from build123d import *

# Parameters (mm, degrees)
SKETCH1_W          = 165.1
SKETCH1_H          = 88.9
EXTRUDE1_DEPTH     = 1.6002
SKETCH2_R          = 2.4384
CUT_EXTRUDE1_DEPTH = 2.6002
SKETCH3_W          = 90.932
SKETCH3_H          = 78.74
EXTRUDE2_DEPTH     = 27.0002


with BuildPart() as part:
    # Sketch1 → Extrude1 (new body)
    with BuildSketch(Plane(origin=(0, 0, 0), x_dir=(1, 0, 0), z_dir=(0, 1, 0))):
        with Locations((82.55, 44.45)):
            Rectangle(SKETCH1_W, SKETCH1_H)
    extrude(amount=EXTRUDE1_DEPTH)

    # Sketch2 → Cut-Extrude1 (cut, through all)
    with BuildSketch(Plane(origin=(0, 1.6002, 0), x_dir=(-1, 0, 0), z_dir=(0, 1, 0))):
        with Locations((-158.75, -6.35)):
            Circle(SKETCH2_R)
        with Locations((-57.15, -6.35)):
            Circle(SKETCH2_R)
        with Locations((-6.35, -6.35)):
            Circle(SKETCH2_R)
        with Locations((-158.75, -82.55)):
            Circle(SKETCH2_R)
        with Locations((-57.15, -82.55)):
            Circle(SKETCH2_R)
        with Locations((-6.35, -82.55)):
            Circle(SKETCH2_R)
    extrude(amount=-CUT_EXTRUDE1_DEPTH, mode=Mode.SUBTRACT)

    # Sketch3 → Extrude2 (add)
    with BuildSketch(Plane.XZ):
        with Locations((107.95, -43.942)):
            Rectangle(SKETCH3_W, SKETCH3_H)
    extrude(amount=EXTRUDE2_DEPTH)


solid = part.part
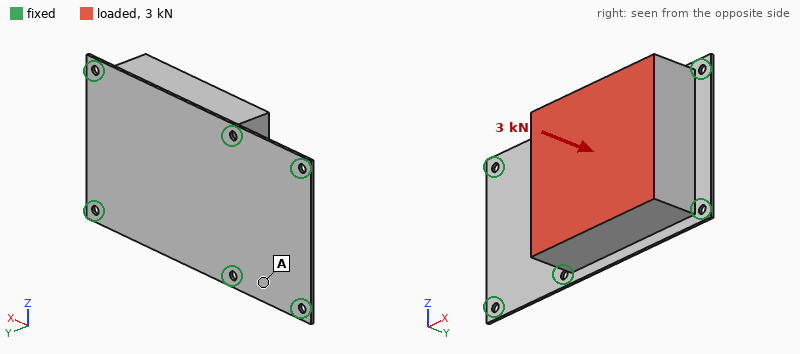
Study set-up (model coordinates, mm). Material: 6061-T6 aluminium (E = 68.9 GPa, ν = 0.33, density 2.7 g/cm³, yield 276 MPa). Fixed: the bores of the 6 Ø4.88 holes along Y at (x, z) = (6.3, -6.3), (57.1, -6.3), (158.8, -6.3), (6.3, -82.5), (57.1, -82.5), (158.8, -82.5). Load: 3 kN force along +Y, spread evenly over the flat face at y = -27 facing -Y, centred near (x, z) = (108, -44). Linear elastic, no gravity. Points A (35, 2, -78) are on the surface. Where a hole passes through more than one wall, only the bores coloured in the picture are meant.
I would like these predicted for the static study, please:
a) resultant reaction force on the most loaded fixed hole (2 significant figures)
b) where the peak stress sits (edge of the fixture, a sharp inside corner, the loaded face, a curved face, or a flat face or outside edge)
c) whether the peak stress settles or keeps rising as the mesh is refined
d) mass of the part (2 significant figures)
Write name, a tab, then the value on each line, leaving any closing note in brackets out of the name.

resultant reaction force on the most loaded fixed hole	920 N
where the peak stress sits	edge of the fixture
whether the peak stress settles or keeps rising as the mesh is refined	keeps rising
mass of the part	580 g
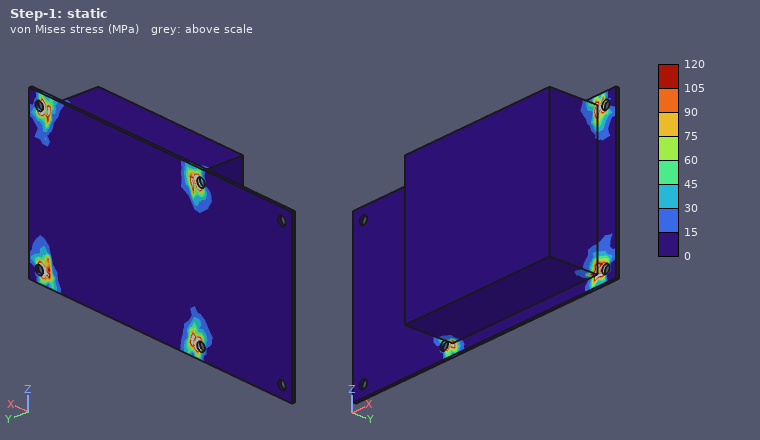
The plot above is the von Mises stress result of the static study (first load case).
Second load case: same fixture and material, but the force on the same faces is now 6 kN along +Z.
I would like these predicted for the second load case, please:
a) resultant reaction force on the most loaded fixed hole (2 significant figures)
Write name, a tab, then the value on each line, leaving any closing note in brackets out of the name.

resultant reaction force on the most loaded fixed hole	2.1 kN
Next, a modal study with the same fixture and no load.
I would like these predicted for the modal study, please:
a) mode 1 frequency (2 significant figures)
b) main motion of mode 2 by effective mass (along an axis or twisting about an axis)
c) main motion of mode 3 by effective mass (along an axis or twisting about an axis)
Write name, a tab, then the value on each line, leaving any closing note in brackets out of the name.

mode 1 frequency	1600 Hz
main motion of mode 2 by effective mass	along Y
main motion of mode 3 by effective mass	along Z
